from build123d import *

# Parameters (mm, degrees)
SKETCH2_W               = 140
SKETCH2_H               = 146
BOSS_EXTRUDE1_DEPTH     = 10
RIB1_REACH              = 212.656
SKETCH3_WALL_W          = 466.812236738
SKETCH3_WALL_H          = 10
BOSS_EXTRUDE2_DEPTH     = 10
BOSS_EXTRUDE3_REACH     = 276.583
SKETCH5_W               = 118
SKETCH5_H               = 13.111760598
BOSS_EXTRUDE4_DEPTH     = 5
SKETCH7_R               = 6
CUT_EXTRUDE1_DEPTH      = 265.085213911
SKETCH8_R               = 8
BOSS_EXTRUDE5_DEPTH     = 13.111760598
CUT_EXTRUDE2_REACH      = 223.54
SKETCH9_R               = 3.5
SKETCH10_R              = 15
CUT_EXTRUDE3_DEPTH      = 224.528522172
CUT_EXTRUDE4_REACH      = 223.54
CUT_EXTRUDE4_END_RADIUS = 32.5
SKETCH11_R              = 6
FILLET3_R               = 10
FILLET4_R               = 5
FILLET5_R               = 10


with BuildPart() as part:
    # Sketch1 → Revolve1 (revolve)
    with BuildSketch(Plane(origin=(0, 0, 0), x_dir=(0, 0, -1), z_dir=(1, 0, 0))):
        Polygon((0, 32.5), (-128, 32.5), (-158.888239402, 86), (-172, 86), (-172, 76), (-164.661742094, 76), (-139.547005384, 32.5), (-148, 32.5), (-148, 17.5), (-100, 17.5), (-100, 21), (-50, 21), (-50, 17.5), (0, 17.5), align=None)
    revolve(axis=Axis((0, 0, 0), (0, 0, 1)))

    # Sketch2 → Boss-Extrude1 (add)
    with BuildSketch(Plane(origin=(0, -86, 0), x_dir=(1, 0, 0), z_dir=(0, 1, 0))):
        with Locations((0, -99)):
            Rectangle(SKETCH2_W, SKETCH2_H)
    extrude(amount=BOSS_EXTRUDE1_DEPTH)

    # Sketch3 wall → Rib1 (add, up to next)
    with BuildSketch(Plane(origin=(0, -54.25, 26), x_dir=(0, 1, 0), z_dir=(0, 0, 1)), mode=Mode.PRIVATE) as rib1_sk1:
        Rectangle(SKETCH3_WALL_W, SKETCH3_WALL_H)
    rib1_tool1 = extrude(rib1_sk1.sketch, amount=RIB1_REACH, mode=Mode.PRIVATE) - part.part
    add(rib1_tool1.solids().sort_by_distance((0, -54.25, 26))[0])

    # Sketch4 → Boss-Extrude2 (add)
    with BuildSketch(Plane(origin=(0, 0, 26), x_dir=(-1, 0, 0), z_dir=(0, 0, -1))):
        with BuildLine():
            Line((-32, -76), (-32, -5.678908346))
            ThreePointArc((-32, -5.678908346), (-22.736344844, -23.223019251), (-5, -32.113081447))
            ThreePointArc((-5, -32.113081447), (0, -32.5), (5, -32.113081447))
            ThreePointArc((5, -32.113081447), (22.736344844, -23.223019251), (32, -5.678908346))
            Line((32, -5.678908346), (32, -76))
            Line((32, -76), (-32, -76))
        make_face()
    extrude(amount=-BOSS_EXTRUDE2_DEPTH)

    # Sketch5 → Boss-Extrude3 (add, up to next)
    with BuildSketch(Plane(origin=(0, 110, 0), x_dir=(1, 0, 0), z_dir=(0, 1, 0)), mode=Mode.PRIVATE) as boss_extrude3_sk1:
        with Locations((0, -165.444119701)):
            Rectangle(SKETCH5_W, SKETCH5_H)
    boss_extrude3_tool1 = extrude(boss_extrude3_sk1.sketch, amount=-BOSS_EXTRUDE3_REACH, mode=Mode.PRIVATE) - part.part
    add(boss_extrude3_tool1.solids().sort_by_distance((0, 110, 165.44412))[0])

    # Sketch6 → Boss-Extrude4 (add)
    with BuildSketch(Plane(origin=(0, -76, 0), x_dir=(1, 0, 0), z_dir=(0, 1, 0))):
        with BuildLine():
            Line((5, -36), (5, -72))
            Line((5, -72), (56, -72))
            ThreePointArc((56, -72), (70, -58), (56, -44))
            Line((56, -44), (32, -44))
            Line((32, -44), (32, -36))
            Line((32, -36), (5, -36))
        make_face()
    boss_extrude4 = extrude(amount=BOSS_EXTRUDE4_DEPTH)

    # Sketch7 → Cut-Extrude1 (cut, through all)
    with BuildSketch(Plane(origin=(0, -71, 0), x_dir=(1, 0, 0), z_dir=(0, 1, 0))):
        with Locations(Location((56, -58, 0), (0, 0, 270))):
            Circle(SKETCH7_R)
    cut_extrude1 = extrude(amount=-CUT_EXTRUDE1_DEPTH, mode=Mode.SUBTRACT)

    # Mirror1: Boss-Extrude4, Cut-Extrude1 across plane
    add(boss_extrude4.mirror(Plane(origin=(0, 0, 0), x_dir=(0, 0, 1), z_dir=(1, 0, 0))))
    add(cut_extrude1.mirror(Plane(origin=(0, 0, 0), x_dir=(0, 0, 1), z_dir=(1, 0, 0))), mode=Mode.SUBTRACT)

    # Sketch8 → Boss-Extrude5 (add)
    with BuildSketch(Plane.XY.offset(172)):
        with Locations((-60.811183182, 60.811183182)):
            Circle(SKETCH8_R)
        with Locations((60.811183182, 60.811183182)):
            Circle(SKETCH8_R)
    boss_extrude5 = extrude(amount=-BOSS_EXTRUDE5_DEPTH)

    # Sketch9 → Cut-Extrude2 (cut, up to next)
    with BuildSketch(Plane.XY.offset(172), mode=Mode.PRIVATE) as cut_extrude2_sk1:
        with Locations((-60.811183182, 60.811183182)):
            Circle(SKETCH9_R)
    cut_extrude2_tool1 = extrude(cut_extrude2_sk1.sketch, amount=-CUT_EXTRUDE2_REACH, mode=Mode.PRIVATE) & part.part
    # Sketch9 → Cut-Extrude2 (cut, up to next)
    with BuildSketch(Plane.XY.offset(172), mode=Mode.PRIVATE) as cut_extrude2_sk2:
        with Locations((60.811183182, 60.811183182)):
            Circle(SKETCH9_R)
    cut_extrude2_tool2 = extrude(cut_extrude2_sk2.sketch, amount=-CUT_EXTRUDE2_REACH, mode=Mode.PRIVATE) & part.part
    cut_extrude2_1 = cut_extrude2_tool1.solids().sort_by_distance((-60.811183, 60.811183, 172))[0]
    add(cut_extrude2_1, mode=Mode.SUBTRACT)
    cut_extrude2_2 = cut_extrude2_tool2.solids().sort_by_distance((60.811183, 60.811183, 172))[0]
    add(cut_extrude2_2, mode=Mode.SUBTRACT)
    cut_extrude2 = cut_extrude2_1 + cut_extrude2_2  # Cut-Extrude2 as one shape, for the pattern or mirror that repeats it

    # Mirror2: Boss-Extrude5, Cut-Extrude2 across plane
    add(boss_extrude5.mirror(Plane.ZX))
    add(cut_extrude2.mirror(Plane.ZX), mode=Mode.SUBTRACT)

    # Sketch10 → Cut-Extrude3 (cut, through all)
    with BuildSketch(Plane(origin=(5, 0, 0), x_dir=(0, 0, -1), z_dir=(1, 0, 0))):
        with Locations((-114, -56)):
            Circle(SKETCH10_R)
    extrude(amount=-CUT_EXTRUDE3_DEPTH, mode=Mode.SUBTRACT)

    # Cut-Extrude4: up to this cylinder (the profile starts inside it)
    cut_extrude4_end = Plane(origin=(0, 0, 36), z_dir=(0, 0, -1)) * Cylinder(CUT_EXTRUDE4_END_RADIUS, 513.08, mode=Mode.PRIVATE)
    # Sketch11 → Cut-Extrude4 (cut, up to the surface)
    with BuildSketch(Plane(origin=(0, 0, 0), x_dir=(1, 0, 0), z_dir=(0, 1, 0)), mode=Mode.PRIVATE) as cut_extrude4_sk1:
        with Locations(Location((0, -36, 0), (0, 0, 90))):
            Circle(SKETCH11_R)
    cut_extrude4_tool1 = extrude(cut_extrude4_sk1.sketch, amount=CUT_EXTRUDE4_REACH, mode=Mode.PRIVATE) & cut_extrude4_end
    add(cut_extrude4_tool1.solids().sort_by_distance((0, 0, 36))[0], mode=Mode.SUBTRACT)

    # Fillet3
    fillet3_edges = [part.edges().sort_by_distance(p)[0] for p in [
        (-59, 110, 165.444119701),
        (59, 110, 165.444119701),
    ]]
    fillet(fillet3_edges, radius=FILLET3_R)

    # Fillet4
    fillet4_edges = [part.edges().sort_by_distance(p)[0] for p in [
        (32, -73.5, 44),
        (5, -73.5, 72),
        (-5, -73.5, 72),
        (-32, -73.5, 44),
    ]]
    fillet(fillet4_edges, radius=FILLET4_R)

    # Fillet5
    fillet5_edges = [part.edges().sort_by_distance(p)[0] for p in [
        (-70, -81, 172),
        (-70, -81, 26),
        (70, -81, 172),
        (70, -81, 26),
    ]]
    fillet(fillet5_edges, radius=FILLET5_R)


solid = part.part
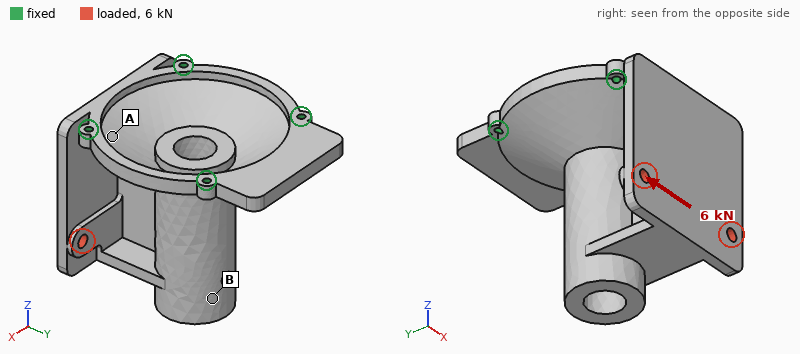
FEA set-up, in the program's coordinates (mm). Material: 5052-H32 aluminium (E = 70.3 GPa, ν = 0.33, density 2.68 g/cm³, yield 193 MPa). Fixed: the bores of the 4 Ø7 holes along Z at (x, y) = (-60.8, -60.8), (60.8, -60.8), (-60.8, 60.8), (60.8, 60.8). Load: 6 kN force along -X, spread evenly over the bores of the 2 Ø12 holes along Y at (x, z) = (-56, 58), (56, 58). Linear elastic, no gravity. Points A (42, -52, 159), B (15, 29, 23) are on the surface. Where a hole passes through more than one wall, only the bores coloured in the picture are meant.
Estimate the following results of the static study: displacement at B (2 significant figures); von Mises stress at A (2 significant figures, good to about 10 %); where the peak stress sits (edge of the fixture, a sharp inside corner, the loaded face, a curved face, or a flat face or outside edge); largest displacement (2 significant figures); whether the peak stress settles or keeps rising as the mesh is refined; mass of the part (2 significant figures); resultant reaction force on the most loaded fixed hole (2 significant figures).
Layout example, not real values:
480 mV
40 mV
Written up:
0.078 mm
13 MPa
edge of the fixture
0.18 mm
keeps rising
2.4 kg
4.7 kN
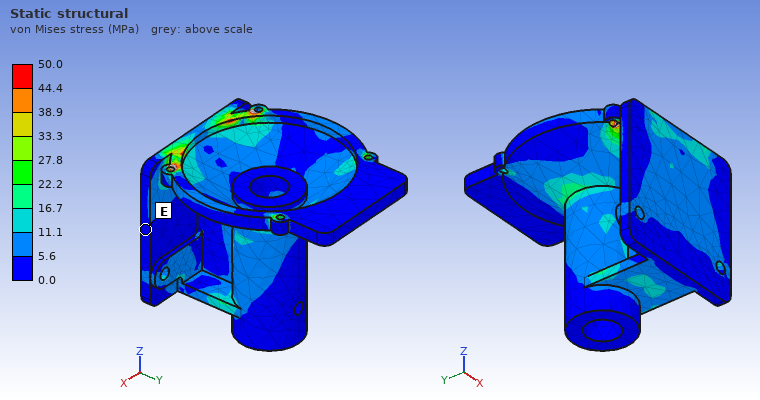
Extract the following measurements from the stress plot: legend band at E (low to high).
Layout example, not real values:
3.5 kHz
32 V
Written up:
0.0 to 5.6 MPa
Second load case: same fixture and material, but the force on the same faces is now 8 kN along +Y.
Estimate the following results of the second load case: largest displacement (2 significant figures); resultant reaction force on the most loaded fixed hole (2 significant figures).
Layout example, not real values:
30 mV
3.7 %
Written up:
0.28 mm
5.6 kN
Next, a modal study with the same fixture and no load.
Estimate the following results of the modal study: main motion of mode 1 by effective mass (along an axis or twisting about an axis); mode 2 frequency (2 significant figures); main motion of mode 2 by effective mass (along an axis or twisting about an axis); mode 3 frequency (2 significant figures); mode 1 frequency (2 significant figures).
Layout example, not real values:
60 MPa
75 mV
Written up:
along X
1300 Hz
along Y
1900 Hz
1100 Hz
